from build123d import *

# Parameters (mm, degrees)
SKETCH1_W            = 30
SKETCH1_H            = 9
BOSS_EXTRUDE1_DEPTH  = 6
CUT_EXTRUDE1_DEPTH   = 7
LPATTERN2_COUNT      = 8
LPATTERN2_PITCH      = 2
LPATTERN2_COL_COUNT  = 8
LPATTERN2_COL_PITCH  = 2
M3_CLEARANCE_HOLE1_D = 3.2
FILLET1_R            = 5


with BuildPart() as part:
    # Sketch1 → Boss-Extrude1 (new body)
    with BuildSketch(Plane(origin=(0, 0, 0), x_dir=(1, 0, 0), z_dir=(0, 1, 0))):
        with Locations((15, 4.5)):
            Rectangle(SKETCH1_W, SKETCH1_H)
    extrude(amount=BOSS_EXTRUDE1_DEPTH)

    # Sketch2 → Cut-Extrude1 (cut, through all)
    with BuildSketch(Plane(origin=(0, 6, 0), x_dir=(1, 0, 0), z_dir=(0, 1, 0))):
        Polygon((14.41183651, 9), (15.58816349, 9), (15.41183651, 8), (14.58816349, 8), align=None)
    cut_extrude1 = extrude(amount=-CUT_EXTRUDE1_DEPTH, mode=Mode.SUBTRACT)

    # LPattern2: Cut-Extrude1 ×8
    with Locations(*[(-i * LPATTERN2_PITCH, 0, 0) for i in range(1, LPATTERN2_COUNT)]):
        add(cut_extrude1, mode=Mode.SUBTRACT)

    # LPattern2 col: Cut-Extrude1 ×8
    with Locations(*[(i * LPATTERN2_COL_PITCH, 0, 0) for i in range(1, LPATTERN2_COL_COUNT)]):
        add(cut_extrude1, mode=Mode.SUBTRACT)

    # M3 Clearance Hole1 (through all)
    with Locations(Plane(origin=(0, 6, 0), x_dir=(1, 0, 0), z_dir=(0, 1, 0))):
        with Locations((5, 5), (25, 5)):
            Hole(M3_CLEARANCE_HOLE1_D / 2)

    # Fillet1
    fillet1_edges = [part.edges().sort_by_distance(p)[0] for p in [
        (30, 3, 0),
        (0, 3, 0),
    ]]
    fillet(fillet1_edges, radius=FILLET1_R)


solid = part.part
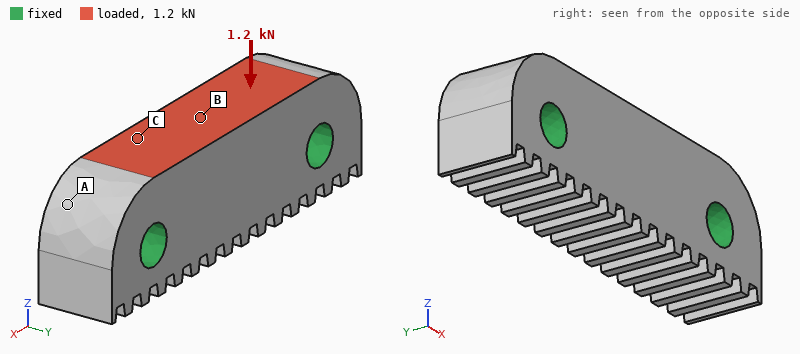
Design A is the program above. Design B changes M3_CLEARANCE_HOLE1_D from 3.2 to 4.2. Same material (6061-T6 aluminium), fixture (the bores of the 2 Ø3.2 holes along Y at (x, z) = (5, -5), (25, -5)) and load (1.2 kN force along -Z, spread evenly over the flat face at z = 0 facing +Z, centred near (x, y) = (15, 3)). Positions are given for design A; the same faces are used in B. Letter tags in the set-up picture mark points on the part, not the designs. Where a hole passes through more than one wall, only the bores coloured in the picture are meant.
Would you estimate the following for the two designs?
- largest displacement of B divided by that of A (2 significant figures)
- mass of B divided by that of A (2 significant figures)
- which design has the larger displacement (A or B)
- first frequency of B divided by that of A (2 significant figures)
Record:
0.82
0.95
A
1.1
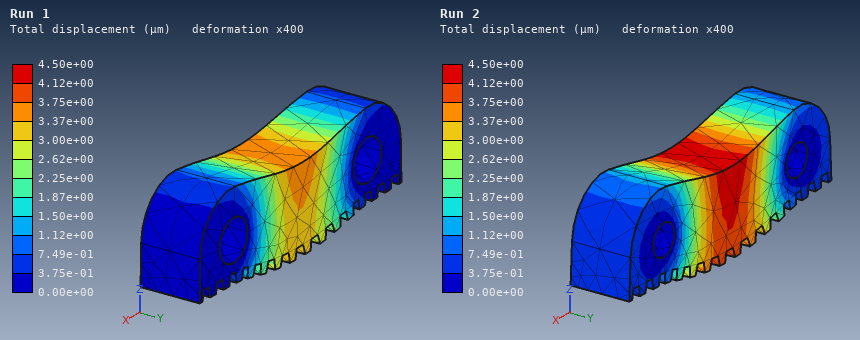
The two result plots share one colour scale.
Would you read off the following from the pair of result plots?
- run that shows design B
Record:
Run 1
